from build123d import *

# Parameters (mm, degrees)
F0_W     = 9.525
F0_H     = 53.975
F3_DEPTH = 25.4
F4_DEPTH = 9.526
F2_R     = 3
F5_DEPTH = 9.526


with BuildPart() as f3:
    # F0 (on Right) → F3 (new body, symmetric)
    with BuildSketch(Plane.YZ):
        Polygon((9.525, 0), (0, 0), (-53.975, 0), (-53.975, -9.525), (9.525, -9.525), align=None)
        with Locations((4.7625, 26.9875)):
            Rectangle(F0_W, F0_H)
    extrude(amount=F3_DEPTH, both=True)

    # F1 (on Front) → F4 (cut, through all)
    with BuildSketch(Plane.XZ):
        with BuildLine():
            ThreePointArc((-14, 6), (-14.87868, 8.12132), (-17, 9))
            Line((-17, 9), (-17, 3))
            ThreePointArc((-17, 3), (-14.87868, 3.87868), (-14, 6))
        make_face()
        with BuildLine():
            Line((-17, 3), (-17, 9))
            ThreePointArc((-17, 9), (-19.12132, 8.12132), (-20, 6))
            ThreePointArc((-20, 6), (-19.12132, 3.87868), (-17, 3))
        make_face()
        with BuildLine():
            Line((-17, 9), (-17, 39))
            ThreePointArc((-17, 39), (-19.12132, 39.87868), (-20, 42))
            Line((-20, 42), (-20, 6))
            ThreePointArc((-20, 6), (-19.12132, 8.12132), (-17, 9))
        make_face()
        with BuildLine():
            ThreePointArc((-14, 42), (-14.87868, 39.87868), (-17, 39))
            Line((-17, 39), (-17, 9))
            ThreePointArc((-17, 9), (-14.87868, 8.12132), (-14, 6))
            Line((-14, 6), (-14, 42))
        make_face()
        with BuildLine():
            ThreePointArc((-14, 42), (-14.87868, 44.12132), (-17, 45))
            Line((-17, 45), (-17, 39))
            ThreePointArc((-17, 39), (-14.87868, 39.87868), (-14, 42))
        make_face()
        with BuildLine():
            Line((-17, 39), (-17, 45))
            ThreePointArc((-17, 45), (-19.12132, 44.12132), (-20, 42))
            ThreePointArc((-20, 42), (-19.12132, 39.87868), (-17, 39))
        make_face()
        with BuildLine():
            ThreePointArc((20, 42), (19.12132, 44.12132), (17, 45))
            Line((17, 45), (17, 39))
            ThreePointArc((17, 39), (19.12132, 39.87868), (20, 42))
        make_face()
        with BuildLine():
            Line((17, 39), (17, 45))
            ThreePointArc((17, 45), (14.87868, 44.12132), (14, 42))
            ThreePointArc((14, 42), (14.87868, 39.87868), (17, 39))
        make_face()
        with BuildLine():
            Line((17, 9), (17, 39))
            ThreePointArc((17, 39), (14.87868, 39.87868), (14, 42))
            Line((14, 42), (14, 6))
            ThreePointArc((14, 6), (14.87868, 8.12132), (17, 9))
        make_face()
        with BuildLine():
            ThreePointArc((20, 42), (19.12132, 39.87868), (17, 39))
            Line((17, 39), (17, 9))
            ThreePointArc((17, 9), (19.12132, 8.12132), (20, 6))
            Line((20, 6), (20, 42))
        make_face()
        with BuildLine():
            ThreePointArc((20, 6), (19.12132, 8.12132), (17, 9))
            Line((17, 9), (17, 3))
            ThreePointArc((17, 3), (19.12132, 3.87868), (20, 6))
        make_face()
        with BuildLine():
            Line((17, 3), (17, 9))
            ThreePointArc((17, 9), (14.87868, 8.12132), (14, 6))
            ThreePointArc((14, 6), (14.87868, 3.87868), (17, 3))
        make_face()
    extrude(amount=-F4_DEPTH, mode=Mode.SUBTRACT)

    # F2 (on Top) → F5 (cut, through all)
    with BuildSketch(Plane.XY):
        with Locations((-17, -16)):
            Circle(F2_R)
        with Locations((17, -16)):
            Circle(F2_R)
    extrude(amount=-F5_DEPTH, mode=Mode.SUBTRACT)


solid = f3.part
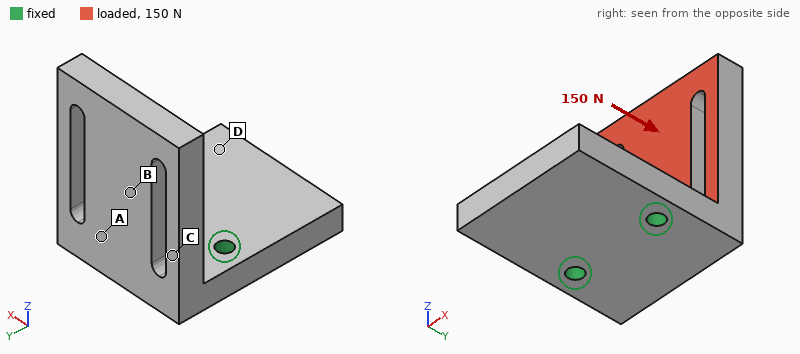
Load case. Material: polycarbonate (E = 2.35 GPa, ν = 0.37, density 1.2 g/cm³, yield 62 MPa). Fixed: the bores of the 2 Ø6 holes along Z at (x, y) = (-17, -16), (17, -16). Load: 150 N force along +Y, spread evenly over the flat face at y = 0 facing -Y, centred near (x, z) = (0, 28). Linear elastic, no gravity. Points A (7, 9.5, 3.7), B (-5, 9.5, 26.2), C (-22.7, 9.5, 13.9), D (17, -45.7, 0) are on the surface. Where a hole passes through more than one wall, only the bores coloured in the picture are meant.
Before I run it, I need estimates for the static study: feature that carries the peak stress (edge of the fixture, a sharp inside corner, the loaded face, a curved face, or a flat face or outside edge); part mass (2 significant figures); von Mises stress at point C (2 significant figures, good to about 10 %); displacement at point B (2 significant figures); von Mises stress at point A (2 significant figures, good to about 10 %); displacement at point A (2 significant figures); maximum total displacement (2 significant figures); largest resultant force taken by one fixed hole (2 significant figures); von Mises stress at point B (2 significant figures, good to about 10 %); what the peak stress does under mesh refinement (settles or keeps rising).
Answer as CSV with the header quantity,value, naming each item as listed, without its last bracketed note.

quantity,value
feature that carries the peak stress,edge of the fixture
part mass,62 g
von Mises stress at point C,4.2 MPa
displacement at point B,0.57 mm
von Mises stress at point A,5.0 MPa
displacement at point A,0.22 mm
maximum total displacement,1.2 mm
largest resultant force taken by one fixed hole,79 N
von Mises stress at point B,1.9 MPa
what the peak stress does under mesh refinement,keeps rising
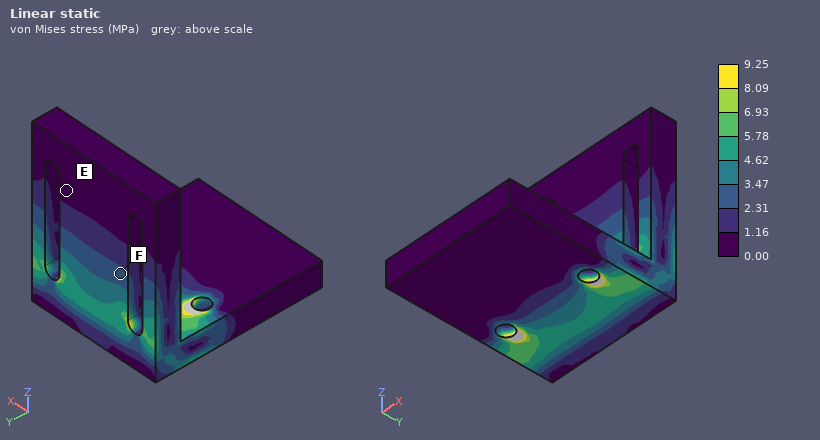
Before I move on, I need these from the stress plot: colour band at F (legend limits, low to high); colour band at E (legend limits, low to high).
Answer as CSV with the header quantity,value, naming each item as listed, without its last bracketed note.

quantity,value
colour band at F,2.31 to 3.47 MPa
colour band at E,0.00 to 1.16 MPa
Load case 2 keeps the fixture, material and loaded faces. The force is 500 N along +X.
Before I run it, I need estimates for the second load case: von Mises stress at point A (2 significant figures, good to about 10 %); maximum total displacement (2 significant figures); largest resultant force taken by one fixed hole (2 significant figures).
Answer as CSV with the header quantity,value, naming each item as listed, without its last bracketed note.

quantity,value
von Mises stress at point A,5.4 MPa
maximum total displacement,1.0 mm
largest resultant force taken by one fixed hole,540 N
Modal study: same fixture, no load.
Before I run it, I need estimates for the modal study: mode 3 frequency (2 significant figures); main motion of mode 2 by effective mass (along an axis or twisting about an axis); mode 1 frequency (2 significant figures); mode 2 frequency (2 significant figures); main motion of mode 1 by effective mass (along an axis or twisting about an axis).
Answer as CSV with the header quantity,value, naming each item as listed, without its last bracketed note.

quantity,value
mode 3 frequency,1300 Hz
main motion of mode 2 by effective mass,along X
mode 1 frequency,420 Hz
mode 2 frequency,850 Hz
main motion of mode 1 by effective mass,along Y
